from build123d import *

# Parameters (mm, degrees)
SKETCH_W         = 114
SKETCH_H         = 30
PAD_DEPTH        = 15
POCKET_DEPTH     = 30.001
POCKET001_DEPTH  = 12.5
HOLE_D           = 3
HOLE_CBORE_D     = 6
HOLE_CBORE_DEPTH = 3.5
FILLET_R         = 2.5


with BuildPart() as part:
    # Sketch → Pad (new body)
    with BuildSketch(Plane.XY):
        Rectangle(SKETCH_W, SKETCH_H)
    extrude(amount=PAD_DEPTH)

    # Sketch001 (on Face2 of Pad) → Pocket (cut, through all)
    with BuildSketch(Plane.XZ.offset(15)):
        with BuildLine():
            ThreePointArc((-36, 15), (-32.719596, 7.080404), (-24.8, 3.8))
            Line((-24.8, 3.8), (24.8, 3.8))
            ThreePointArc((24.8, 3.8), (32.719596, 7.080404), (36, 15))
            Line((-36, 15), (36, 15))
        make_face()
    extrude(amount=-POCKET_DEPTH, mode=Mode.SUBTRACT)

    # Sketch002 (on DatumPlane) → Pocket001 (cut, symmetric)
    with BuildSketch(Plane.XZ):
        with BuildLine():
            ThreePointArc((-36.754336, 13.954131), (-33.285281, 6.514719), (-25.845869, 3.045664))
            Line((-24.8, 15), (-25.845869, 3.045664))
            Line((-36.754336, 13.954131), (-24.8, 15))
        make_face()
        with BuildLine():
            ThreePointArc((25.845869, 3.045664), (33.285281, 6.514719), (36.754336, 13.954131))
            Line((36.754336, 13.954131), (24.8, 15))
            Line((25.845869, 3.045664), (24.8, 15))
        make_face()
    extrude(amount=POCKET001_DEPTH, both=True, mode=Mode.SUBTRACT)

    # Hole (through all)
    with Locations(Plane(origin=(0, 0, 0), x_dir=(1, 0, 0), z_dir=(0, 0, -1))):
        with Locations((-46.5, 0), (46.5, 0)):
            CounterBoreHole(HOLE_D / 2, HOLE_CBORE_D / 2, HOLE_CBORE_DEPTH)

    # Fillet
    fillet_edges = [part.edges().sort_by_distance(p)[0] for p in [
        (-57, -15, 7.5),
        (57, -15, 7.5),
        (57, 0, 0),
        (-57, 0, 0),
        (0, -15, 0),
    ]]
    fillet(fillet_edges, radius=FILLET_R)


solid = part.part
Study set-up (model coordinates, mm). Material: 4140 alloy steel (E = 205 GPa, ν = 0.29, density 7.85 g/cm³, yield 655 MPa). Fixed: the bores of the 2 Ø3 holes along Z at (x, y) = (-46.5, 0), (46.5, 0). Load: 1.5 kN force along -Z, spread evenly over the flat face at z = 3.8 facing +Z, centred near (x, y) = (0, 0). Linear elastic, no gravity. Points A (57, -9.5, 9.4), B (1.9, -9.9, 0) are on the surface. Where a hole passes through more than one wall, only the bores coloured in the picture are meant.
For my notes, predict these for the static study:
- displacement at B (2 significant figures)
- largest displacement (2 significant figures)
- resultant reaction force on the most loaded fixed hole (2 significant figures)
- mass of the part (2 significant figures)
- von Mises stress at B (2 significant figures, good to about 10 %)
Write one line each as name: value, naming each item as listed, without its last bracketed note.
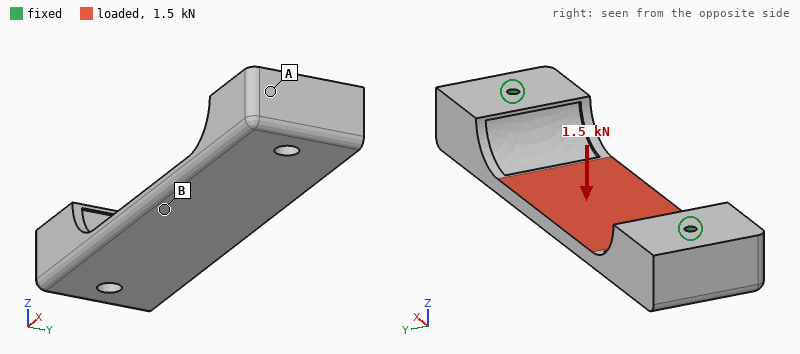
displacement at B: 59 µm
largest displacement: 62 µm
resultant reaction force on the most loaded fixed hole: 1.2 kN
mass of the part: 220 g
von Mises stress at B: 87 MPa
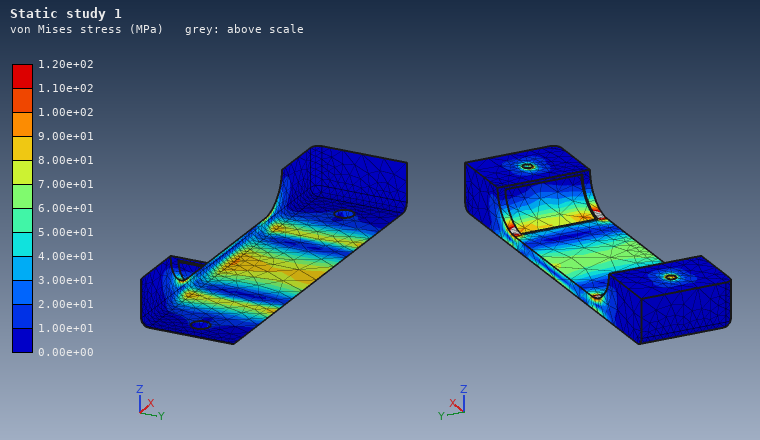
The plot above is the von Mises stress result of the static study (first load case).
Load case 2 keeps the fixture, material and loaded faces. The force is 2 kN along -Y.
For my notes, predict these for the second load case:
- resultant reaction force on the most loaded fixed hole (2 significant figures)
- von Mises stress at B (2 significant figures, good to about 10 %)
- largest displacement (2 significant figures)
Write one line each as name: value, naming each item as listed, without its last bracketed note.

resultant reaction force on the most loaded fixed hole: 1.0 kN
von Mises stress at B: 37 MPa
largest displacement: 18 µm
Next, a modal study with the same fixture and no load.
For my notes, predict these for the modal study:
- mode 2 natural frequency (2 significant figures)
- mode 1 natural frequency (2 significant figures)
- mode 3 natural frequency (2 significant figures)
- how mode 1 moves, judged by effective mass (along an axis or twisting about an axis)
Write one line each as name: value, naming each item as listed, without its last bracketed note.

mode 2 natural frequency: 7100 Hz
mode 1 natural frequency: 4300 Hz
mode 3 natural frequency: 7800 Hz
how mode 1 moves, judged by effective mass: along Z
